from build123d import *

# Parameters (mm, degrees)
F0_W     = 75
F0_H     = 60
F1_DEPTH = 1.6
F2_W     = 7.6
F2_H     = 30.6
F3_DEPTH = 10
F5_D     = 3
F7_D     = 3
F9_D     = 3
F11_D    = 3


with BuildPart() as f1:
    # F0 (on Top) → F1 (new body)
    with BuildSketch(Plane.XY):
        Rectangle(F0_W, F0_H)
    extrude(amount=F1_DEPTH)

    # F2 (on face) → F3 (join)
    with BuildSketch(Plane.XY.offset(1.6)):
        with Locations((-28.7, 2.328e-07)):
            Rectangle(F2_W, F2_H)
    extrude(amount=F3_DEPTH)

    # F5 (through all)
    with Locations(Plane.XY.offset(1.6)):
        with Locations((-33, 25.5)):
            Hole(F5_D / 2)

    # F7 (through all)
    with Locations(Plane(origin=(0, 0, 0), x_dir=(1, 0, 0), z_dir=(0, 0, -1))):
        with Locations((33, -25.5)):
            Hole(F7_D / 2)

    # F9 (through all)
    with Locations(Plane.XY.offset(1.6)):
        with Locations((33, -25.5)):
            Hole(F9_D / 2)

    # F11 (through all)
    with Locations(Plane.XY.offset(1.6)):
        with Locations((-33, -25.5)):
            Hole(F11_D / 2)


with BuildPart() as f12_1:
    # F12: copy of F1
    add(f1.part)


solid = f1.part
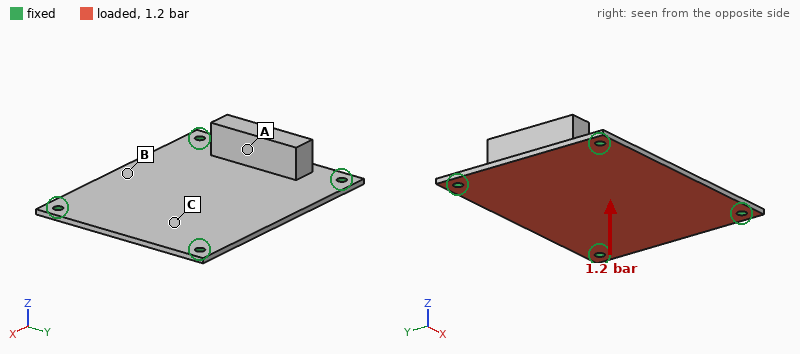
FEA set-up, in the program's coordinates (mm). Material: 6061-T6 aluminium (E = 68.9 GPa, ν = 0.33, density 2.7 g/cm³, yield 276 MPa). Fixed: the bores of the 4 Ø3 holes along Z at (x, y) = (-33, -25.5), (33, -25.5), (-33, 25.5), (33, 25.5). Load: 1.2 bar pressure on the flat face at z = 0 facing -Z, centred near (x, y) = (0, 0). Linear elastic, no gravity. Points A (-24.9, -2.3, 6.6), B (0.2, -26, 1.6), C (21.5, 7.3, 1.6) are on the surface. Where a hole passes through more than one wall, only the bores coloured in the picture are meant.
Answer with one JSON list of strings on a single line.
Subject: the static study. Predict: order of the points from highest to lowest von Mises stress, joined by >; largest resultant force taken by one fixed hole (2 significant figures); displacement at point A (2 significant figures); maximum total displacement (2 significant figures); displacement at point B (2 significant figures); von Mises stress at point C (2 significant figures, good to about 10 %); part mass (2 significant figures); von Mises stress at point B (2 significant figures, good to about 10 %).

["B > C > A", "140 N", "0.14 mm", "0.39 mm", "0.34 mm", "32 MPa", "26 g", "64 MPa"]
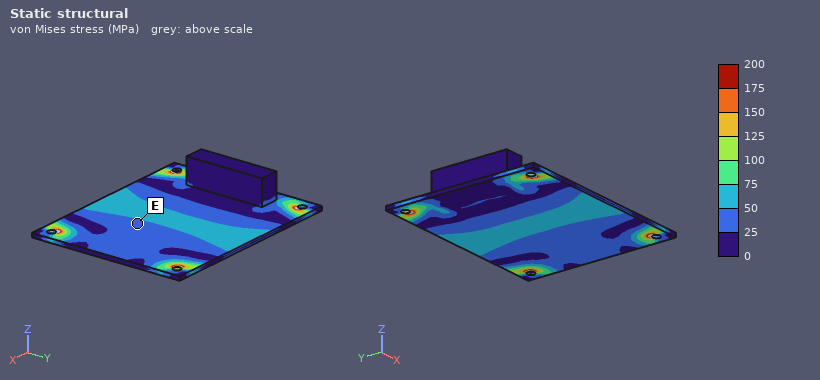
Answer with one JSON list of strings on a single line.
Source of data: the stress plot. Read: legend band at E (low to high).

["25 to 50 MPa"]
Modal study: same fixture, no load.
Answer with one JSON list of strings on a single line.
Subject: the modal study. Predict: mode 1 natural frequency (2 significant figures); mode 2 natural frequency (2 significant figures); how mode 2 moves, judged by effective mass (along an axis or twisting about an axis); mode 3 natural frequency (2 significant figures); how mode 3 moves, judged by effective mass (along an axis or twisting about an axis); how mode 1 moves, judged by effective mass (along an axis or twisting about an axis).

["1500 Hz", "2600 Hz", "twisting about X", "3200 Hz", "twisting about Y", "along Z"]
